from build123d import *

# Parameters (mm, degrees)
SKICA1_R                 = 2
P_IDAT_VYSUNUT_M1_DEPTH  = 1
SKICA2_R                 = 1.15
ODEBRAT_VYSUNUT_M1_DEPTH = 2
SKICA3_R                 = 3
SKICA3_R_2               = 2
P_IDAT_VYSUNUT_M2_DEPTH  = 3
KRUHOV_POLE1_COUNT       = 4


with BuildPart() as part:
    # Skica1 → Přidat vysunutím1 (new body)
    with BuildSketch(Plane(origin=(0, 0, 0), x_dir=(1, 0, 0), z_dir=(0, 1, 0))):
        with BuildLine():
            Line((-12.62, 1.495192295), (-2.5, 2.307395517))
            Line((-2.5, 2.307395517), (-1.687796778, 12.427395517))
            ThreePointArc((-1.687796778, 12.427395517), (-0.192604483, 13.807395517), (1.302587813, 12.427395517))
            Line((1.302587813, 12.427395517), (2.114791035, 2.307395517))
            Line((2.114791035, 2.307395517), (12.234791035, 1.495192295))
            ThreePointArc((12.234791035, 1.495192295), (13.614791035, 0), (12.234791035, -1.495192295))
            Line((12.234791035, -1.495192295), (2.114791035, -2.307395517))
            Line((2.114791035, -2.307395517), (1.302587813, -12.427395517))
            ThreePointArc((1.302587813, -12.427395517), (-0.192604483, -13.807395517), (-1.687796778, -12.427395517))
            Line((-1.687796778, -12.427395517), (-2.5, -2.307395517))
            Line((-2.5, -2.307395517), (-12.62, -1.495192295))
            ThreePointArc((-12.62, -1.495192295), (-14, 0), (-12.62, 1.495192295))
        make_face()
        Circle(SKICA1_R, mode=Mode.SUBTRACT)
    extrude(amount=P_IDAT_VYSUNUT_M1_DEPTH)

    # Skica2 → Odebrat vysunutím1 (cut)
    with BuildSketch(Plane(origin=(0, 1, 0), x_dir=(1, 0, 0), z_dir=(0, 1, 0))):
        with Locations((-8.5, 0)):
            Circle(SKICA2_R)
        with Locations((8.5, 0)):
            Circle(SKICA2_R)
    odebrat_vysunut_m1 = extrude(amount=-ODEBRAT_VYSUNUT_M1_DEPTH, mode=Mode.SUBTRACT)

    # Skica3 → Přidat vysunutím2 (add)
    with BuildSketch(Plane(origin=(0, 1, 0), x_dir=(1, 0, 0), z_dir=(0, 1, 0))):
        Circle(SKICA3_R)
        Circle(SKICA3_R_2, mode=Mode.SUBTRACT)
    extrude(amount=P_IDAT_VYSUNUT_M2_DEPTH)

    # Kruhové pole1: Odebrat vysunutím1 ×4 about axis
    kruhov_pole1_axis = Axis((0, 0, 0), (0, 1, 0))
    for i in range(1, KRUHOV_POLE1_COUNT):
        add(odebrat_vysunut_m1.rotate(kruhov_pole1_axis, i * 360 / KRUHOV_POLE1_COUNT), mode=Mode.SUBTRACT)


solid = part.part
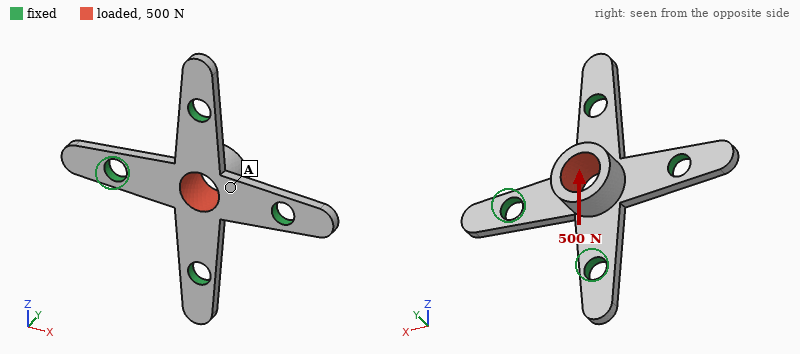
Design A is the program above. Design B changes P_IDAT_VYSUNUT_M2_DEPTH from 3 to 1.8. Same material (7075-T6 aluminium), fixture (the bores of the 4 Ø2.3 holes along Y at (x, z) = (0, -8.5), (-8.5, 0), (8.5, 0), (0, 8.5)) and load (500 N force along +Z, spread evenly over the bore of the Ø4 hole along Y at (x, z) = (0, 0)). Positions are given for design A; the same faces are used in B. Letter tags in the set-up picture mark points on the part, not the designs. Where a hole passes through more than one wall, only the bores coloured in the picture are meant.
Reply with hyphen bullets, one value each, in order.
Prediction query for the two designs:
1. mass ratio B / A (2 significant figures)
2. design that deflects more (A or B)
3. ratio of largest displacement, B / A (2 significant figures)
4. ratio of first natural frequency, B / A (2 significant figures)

- 0.91
- A
- 0.50
- 1.1
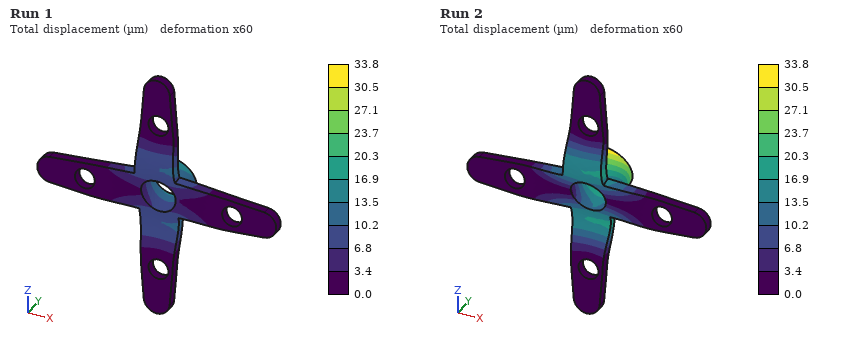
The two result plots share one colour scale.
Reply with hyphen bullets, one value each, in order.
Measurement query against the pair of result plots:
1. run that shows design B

- Run 1
